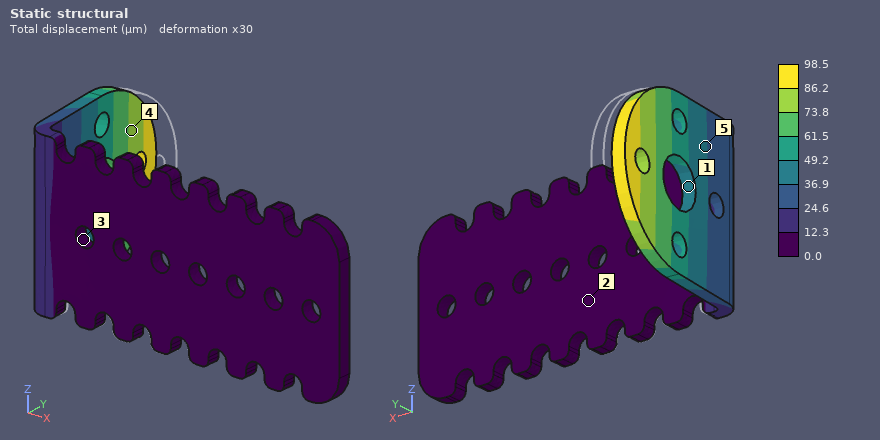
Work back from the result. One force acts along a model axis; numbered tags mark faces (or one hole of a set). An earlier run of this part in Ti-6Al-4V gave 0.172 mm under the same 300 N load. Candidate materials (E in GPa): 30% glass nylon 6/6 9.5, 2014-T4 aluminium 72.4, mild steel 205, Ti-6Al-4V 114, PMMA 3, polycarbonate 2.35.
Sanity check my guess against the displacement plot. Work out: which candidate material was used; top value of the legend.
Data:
mild steel
98.5 µm
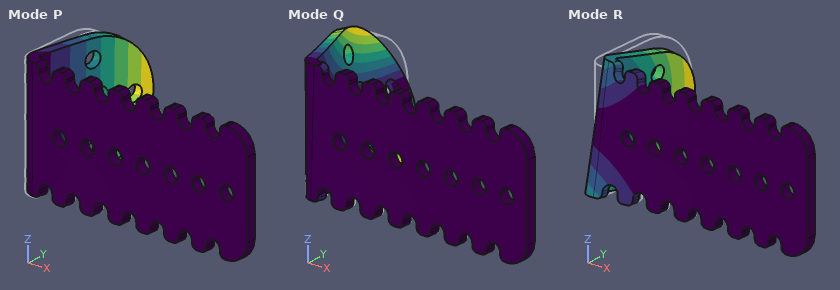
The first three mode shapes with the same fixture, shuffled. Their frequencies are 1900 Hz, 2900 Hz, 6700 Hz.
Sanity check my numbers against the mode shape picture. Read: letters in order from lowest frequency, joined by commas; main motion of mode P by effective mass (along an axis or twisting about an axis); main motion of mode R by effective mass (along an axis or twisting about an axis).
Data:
P, R, Q
along X
along Z
